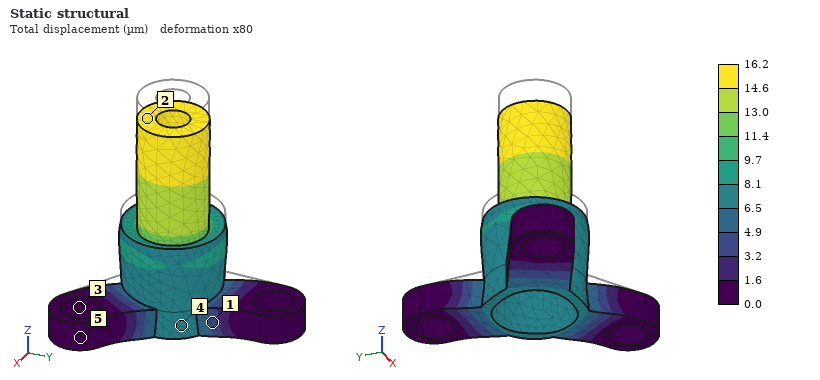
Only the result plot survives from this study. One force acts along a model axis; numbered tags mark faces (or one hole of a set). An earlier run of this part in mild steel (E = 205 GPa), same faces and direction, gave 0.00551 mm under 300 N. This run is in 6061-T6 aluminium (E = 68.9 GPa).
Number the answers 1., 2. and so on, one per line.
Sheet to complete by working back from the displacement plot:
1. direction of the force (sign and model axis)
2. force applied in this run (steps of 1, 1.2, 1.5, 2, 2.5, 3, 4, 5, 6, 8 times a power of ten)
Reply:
1. -Z
2. 300 N
